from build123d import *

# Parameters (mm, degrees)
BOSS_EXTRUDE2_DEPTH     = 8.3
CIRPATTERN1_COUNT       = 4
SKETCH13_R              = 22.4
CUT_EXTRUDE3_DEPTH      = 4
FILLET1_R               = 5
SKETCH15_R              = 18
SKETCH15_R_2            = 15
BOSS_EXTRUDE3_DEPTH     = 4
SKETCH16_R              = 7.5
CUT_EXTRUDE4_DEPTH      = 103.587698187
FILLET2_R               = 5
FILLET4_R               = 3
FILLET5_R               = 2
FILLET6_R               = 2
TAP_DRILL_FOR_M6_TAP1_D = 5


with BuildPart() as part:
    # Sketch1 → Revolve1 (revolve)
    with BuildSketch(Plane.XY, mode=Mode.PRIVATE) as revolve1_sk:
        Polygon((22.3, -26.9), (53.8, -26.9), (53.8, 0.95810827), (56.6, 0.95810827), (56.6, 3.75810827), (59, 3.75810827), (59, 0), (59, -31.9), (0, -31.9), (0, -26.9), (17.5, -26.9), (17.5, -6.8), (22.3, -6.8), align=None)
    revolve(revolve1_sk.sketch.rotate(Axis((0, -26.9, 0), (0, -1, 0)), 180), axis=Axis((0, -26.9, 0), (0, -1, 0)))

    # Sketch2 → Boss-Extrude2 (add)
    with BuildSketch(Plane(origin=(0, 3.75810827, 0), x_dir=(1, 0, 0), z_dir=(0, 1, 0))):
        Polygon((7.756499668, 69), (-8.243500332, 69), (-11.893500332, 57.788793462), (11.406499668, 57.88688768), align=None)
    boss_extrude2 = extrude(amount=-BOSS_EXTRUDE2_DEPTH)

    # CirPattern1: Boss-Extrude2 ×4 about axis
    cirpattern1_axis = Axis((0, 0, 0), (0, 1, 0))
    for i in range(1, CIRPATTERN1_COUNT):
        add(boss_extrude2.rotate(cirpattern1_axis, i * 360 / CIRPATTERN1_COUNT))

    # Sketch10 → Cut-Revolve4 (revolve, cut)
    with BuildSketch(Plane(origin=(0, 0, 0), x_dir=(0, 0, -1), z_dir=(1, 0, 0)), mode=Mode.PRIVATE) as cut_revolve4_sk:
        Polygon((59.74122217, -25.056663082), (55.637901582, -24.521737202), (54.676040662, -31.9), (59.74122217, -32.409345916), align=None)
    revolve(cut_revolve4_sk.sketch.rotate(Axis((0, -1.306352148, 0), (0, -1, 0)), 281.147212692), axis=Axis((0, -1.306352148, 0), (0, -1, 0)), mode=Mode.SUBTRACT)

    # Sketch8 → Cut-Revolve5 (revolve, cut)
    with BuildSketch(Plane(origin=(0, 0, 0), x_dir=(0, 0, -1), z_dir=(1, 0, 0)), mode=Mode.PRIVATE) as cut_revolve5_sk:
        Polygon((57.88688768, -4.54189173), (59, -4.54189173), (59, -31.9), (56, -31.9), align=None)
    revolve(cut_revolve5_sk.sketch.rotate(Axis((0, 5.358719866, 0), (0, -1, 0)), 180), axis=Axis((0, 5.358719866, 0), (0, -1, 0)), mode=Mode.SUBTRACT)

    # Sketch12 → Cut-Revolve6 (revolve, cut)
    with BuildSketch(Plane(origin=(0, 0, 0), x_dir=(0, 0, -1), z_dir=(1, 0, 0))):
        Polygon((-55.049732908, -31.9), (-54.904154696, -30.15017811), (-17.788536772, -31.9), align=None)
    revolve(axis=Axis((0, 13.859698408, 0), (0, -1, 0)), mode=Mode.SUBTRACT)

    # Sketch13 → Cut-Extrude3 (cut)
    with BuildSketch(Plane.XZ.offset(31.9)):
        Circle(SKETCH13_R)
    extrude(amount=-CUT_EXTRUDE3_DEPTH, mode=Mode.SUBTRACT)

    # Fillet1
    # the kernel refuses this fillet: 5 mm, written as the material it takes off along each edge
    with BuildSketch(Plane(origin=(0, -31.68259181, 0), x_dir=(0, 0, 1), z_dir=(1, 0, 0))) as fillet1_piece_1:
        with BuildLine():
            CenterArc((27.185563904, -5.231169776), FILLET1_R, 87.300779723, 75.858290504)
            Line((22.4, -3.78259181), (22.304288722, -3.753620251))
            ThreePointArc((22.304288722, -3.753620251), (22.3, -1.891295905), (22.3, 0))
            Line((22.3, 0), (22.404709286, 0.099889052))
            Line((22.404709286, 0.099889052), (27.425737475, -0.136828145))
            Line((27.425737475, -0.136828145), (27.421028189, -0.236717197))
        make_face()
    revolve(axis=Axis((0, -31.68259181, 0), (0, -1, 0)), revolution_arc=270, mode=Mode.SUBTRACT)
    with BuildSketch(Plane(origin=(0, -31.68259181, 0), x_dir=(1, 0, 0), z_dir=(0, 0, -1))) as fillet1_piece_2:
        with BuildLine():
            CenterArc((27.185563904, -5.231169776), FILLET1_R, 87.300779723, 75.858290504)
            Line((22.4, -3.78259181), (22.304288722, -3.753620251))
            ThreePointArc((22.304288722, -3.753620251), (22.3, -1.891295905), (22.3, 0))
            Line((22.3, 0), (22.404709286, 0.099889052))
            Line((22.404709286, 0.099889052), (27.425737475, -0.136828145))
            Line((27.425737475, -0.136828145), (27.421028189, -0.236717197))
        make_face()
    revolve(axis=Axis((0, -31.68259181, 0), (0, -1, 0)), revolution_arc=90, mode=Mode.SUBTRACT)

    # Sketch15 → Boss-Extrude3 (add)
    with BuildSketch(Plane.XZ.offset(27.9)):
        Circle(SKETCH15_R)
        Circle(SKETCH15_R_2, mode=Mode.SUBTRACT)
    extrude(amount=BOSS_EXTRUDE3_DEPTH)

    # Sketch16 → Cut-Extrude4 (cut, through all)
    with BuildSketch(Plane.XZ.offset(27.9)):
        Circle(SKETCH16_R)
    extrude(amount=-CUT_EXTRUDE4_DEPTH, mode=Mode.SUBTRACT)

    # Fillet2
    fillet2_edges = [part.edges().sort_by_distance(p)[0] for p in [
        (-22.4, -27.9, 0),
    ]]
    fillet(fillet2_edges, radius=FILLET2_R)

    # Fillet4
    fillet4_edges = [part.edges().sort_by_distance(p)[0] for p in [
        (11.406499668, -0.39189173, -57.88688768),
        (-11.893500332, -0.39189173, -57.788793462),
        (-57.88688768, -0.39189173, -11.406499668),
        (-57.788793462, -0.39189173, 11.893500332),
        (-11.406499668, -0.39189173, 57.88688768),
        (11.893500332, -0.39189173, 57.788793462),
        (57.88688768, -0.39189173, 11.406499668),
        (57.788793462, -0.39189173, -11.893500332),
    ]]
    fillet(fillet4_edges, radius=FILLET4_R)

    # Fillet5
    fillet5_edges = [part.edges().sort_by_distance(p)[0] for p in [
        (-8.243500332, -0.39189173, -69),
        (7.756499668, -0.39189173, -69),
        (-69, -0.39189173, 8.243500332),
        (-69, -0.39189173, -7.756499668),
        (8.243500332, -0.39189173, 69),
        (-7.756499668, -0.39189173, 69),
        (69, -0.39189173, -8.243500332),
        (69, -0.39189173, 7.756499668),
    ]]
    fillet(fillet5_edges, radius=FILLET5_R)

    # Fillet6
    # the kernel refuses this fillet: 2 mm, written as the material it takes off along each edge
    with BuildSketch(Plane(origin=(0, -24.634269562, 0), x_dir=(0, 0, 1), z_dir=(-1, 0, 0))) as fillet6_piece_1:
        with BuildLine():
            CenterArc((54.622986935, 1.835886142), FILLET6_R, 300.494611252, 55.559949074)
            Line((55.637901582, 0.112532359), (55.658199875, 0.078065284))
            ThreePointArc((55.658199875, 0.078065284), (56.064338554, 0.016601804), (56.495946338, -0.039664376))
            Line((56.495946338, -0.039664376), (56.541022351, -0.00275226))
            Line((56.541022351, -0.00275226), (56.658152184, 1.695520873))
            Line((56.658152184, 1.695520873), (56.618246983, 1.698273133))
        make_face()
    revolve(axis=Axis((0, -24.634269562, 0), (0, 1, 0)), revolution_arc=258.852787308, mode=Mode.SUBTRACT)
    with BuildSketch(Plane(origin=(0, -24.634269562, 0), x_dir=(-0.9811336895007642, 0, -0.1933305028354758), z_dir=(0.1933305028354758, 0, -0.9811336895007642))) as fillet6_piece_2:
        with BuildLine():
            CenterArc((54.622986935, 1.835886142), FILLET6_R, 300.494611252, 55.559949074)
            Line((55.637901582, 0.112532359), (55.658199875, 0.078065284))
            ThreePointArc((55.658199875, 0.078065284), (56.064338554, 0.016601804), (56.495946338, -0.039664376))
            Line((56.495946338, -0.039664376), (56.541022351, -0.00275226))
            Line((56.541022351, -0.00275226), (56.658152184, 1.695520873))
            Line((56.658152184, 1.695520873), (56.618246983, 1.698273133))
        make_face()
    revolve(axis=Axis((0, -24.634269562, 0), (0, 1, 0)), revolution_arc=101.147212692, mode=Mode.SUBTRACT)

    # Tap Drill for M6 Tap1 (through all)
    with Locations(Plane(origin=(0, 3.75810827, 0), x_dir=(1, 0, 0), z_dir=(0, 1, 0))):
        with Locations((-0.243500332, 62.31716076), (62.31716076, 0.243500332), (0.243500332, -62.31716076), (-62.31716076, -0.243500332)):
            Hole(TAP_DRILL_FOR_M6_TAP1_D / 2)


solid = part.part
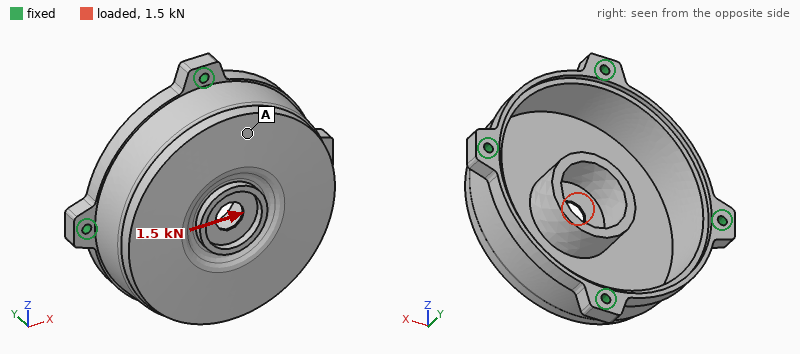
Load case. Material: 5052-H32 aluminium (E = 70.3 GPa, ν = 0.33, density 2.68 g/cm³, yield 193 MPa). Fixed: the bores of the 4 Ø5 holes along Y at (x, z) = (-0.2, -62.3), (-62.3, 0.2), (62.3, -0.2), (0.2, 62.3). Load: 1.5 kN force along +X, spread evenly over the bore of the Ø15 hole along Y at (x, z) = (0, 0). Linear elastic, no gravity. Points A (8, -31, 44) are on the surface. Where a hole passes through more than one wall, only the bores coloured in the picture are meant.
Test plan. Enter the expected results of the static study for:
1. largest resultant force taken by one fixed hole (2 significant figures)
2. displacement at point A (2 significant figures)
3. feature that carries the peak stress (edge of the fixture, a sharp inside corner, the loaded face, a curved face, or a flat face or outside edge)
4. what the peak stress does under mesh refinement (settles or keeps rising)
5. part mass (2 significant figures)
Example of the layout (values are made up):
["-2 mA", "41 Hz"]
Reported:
["530 N", "7.0 µm", "a sharp inside corner", "keeps rising", "240 g"]
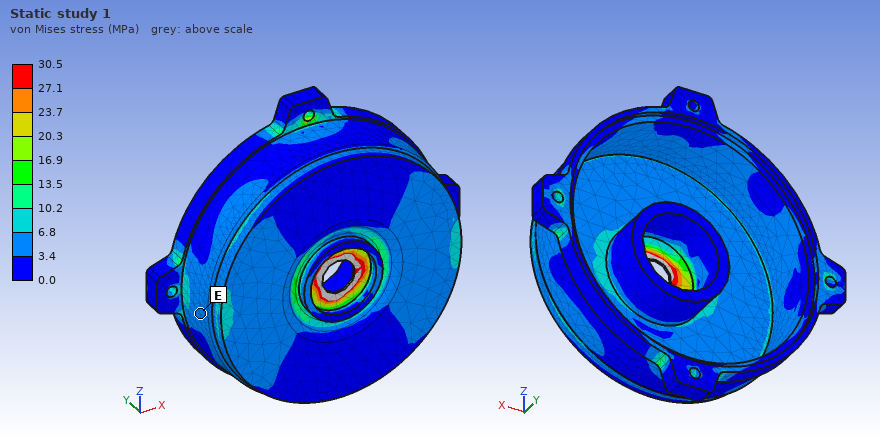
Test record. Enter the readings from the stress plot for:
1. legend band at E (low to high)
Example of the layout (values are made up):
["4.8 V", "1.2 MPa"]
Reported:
["3.4 to 6.8 MPa"]
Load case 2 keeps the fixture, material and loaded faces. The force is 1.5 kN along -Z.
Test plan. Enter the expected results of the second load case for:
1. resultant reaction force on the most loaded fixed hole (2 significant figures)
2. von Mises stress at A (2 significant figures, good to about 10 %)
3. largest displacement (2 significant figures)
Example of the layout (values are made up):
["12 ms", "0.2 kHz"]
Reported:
["530 N", "6.0 MPa", "16 µm"]
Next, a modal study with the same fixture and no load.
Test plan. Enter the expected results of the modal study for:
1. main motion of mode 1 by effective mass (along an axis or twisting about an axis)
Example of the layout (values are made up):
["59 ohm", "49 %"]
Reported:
["along Y"]
